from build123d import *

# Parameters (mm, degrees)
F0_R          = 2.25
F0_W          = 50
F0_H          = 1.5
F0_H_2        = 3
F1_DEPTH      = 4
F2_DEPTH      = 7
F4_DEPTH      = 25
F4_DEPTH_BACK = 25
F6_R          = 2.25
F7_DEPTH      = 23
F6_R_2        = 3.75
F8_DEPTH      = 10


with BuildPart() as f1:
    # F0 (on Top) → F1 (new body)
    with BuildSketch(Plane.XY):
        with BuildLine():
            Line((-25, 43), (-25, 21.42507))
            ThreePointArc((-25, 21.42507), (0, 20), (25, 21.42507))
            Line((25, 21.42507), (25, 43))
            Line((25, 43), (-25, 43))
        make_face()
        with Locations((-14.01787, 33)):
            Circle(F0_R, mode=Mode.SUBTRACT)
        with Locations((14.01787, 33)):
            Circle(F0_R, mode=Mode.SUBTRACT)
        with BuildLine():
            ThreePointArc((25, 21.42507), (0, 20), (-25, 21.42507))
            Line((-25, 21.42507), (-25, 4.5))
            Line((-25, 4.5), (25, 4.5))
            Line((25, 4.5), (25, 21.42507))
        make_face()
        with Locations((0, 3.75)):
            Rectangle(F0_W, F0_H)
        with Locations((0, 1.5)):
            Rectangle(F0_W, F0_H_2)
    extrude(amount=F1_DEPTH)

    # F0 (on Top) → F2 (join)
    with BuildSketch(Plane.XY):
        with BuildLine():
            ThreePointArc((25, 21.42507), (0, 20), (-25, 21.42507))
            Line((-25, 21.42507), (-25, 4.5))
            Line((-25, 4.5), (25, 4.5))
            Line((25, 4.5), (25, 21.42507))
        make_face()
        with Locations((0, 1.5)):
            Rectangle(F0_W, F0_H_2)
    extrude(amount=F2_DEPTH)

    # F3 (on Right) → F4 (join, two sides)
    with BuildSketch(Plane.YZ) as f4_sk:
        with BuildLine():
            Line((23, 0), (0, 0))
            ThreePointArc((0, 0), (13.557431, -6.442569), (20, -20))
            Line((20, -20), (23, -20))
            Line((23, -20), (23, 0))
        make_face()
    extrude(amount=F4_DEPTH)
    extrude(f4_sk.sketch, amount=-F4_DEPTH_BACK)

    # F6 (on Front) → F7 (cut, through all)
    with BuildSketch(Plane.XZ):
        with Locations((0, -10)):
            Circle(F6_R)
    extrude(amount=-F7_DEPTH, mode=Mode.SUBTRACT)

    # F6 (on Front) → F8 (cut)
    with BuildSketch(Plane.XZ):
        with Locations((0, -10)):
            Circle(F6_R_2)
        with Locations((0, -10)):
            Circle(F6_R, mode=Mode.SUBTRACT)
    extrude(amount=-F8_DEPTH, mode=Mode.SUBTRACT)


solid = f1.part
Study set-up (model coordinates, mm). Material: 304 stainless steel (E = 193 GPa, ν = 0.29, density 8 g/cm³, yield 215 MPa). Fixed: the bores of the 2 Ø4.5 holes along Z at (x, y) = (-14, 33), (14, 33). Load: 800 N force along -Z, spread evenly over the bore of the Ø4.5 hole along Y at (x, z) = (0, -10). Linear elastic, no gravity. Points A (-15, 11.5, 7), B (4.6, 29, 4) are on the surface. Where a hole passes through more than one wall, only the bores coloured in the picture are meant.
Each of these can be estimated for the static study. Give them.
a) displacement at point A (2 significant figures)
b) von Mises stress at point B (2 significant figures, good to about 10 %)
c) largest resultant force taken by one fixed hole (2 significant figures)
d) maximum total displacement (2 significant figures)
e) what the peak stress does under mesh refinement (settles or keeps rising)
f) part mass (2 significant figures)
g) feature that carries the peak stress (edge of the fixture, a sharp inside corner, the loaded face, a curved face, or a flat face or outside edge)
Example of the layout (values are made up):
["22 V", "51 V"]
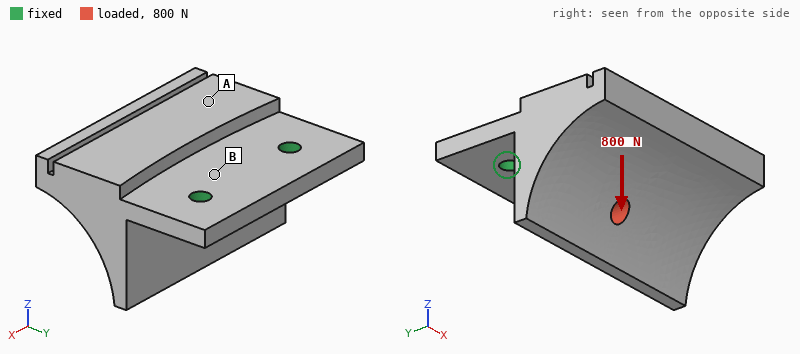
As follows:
["27 µm", "34 MPa", "400 N", "43 µm", "keeps rising", "150 g", "edge of the fixture"]
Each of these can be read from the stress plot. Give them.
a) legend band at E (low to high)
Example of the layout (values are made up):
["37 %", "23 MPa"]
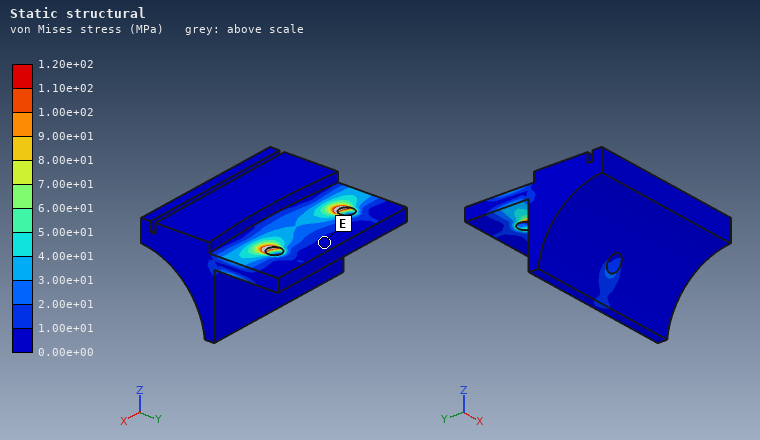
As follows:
["0.00e+00 to 1.00e+01 MPa"]
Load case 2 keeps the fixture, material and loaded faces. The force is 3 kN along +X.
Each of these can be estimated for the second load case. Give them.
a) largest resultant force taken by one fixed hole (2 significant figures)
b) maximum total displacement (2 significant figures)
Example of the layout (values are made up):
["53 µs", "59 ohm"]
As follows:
["2.2 kN", "29 µm"]
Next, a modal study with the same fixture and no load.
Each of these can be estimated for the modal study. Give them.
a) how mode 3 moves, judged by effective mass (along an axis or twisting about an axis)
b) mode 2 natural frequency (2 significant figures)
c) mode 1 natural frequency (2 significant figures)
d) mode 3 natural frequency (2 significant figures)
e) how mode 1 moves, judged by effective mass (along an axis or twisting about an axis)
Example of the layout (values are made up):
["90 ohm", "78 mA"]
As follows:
["along X", "5500 Hz", "1800 Hz", "9800 Hz", "along Z"]
